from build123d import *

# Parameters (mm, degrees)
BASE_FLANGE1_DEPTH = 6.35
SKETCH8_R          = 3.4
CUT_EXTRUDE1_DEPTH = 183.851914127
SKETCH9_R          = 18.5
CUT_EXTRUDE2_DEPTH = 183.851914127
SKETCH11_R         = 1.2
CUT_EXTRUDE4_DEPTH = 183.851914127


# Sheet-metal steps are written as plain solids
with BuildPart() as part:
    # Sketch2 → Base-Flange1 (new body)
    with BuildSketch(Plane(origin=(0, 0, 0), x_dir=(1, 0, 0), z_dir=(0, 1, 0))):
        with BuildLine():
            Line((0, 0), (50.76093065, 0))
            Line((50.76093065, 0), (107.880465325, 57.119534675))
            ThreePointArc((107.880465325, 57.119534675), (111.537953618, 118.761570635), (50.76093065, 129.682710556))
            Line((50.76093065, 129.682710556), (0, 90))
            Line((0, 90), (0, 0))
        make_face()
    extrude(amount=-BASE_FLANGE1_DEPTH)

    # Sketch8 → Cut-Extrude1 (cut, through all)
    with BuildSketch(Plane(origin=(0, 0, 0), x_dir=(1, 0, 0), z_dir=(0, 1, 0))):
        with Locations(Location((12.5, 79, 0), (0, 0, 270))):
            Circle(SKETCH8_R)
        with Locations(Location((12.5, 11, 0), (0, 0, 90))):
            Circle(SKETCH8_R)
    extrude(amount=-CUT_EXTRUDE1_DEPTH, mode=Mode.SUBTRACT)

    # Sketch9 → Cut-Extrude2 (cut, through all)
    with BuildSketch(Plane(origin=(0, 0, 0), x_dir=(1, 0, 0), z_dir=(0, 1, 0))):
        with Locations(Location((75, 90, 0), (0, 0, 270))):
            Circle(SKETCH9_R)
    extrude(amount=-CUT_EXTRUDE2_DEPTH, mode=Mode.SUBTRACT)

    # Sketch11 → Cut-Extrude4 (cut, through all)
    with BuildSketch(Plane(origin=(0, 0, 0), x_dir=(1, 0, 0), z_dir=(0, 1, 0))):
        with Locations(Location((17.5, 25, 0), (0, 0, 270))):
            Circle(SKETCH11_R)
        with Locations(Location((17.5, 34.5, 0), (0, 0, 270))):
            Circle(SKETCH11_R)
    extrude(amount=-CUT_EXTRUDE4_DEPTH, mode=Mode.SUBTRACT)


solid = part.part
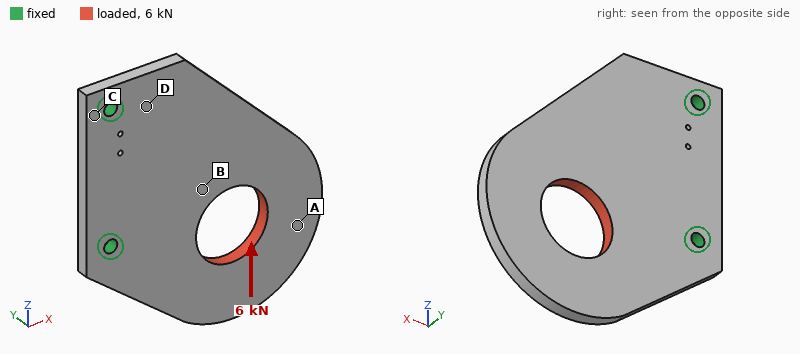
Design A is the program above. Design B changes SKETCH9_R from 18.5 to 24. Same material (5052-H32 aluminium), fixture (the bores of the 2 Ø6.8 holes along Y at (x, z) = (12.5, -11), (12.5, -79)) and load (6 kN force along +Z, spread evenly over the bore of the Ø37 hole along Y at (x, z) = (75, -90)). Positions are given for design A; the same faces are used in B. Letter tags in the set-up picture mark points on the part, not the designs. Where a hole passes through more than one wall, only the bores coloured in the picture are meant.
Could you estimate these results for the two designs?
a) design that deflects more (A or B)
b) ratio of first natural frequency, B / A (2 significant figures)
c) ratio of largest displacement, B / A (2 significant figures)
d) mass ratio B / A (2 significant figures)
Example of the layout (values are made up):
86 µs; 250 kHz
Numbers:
B; 1.0; 1.2; 0.93
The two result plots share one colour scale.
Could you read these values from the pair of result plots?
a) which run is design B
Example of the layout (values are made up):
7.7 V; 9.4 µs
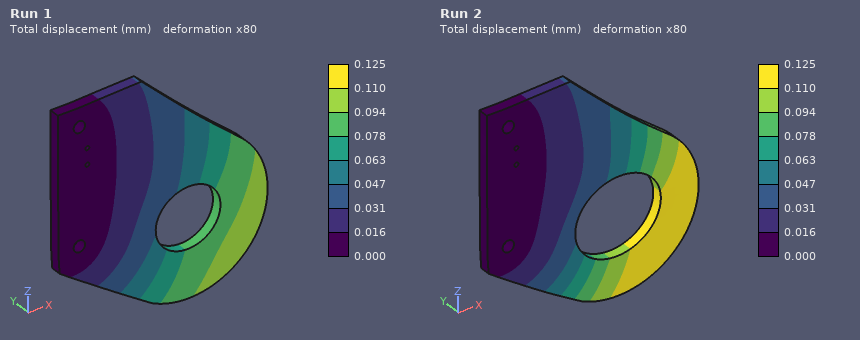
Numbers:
Run 2
